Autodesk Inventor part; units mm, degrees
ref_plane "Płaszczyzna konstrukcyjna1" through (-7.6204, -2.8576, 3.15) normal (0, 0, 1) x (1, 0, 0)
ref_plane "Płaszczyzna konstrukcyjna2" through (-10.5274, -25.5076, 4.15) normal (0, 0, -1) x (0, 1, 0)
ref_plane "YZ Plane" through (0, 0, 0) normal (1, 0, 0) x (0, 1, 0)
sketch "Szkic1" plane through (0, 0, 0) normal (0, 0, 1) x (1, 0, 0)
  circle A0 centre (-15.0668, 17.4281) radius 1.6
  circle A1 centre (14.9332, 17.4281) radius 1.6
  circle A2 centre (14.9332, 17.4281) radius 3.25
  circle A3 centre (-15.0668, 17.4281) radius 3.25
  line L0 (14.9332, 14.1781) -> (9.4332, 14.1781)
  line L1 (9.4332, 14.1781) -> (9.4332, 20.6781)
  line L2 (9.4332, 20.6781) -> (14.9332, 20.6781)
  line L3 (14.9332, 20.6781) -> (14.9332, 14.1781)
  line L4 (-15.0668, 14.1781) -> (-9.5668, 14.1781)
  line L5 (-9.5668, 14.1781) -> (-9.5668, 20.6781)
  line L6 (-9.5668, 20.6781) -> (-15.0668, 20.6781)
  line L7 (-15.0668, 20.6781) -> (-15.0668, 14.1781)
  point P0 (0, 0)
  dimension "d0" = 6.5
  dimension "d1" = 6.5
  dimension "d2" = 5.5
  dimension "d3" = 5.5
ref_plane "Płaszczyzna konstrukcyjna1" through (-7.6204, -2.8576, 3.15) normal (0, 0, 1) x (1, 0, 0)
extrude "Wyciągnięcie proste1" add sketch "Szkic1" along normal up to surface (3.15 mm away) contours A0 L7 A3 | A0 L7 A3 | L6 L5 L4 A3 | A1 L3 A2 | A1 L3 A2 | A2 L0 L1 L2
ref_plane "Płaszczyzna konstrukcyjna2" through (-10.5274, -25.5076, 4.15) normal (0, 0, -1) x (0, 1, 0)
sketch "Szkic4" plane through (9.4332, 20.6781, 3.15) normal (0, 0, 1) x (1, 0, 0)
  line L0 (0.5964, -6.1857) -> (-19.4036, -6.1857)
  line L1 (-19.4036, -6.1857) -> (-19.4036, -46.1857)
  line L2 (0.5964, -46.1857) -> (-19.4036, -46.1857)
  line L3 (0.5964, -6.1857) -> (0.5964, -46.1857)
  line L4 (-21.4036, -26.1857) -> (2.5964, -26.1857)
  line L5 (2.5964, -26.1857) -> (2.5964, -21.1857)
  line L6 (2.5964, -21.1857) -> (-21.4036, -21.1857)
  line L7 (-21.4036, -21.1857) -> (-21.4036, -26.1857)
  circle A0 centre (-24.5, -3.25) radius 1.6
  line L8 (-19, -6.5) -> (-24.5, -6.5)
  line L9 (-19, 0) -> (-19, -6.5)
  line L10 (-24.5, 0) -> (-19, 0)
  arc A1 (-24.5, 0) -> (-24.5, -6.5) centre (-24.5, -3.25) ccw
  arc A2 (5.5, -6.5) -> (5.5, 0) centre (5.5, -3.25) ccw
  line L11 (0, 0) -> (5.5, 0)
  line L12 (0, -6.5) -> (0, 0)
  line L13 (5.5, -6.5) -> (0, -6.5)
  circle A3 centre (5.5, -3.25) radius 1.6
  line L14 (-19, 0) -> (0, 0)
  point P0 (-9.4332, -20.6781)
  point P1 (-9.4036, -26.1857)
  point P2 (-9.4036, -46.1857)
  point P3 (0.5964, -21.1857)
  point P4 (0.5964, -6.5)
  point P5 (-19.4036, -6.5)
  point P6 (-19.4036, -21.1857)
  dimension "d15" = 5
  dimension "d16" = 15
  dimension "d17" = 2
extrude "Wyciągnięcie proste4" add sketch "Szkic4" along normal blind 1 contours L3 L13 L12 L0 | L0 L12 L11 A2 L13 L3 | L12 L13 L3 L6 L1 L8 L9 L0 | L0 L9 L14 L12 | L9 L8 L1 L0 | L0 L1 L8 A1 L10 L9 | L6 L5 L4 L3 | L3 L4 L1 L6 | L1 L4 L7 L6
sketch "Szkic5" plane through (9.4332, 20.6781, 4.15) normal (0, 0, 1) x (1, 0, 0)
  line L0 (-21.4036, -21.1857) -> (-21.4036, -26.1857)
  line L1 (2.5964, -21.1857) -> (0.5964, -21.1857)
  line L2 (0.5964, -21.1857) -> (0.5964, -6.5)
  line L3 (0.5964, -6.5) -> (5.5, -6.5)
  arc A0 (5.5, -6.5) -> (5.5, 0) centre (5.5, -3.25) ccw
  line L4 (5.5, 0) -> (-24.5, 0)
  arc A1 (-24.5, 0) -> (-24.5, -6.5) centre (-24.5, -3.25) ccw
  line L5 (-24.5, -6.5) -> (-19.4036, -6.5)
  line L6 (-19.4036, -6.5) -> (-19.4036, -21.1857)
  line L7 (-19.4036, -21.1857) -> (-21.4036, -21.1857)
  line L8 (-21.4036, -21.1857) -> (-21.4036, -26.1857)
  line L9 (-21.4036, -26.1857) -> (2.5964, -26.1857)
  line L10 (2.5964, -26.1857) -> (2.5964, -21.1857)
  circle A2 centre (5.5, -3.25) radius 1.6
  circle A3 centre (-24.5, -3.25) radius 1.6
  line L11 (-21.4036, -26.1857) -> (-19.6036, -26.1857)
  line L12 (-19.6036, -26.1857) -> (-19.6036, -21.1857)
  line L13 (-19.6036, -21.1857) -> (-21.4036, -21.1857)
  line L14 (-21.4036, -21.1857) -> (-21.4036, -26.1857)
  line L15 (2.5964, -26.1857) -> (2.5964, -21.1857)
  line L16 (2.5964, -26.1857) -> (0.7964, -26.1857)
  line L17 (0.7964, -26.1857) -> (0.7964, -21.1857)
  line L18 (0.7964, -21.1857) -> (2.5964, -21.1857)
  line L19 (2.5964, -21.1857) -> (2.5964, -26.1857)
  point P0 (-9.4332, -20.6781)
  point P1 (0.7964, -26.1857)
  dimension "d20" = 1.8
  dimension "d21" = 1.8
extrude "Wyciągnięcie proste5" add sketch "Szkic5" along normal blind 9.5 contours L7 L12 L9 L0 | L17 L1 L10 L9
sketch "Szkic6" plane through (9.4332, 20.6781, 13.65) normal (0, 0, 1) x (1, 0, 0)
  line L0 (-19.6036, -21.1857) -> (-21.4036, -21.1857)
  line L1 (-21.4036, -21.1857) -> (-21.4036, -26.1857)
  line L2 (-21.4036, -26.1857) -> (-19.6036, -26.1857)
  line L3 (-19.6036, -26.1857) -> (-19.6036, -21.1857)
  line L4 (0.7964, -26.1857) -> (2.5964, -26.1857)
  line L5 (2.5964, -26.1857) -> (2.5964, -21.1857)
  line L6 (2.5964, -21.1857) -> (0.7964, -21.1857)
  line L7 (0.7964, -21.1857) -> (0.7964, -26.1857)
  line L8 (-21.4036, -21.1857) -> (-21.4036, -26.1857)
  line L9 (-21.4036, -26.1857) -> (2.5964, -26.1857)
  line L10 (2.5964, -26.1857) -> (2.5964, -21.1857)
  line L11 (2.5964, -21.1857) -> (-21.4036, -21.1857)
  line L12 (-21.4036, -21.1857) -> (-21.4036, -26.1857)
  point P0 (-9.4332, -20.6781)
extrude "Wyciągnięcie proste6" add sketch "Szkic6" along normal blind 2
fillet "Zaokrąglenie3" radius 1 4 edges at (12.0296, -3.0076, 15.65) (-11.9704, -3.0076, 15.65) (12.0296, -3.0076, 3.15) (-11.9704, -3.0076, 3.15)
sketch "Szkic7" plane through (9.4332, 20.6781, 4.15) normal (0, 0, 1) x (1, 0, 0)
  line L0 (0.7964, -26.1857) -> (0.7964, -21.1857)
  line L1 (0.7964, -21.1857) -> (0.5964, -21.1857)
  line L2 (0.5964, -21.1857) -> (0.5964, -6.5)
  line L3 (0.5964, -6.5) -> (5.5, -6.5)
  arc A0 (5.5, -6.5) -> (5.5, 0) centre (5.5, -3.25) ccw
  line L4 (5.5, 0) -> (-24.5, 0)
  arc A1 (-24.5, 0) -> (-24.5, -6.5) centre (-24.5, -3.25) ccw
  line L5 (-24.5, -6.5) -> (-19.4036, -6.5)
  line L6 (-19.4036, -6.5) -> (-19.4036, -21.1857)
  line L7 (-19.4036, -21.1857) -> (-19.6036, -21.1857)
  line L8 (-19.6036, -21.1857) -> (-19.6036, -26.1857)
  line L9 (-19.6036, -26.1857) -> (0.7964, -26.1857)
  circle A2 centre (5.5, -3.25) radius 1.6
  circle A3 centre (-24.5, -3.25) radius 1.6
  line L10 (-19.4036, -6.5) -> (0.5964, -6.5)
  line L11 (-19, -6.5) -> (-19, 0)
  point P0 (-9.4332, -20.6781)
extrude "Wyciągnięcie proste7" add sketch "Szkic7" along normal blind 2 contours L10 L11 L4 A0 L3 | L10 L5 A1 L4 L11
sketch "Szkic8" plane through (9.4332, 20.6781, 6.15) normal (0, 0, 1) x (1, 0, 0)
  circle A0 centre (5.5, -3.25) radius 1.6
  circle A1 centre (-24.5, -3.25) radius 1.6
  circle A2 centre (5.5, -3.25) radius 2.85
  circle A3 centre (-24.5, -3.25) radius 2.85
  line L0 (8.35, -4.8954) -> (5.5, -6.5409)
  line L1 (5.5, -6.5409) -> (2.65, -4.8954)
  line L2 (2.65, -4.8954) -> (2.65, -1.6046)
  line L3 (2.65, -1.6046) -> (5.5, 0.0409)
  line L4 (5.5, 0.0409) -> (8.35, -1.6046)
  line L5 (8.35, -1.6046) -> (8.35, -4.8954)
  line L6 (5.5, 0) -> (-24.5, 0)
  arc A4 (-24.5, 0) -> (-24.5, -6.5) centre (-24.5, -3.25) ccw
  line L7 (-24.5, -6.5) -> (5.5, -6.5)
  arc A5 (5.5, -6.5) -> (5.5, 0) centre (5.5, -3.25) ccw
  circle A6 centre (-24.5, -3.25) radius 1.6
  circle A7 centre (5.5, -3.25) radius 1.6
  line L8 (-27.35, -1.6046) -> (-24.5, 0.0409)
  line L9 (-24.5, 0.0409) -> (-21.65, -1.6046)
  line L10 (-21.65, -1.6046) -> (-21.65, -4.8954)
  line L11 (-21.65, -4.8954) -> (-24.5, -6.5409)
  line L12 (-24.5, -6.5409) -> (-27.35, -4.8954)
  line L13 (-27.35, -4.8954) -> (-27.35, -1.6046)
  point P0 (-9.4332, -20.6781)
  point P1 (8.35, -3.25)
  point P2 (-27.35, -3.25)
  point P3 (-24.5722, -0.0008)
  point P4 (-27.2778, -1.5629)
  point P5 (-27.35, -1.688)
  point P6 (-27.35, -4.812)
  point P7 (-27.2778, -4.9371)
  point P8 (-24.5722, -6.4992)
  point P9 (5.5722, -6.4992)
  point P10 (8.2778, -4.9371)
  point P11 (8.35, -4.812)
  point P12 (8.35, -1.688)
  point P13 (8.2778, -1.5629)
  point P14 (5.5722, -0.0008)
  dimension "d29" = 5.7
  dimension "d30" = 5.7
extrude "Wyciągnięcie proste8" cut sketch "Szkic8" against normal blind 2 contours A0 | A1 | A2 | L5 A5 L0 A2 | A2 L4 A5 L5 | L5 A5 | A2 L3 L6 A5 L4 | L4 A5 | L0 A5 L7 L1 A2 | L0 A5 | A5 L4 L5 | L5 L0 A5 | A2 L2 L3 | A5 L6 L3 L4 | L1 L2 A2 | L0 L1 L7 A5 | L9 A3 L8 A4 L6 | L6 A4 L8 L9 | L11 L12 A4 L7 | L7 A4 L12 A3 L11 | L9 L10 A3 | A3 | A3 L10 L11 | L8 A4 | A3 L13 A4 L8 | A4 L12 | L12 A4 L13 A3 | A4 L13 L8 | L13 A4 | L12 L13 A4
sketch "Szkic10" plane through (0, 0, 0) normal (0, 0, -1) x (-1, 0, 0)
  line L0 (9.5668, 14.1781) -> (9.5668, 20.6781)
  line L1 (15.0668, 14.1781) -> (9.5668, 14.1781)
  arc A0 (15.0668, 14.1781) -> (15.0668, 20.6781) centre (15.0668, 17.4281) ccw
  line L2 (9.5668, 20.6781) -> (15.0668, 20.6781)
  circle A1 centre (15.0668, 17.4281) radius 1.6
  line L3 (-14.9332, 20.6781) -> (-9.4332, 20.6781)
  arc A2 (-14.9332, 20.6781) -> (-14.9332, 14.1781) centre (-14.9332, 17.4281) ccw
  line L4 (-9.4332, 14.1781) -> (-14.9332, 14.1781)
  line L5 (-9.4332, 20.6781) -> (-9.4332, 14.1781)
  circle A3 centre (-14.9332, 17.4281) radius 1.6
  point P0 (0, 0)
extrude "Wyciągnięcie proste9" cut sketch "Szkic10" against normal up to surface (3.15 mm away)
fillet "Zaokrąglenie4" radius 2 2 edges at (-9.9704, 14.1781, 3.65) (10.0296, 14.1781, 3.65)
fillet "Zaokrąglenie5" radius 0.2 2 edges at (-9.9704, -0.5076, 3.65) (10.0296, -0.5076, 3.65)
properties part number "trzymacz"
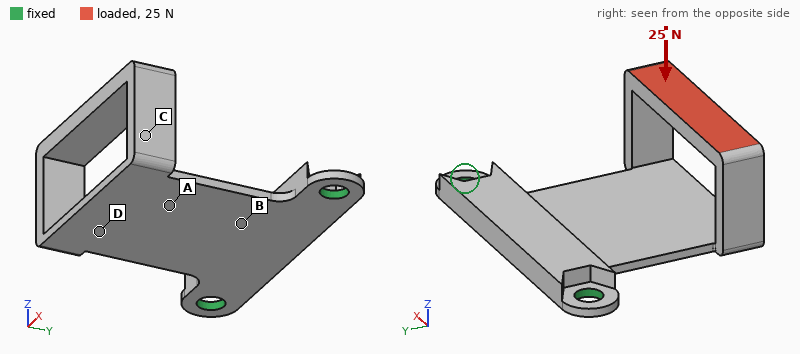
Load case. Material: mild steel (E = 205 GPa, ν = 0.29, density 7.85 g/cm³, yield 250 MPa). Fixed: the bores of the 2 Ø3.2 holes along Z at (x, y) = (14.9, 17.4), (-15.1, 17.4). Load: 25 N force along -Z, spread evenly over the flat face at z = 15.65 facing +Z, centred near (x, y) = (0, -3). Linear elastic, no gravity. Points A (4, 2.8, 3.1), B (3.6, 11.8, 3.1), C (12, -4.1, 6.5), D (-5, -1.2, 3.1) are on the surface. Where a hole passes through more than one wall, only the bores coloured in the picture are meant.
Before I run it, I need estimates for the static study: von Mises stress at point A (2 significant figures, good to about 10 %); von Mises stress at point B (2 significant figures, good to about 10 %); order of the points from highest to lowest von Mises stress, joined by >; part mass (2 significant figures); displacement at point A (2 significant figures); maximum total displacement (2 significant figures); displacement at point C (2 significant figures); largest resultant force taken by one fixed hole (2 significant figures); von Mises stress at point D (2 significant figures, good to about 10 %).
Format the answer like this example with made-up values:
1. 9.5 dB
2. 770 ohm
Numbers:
1. 39 MPa
2. 98 MPa
3. B > A > D > C
4. 11 g
5. 0.087 mm
6. 0.24 mm
7. 0.18 mm
8. 42 N
9. 18 MPa
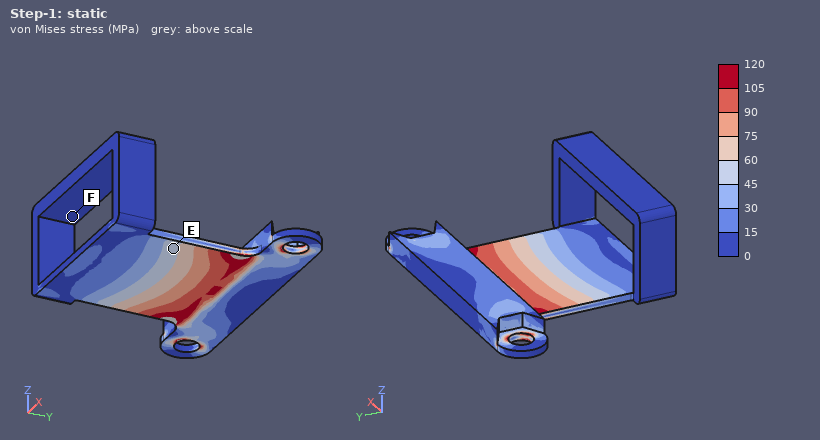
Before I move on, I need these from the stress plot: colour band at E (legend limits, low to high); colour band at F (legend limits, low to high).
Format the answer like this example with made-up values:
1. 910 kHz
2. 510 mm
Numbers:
1. 45 to 60 MPa
2. 0 to 15 MPa
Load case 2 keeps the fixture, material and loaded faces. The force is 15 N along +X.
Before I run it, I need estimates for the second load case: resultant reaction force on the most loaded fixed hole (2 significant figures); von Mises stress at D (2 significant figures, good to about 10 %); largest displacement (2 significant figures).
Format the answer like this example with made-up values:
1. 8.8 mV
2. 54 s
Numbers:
1. 15 N
2. 19 MPa
3. 62 µm
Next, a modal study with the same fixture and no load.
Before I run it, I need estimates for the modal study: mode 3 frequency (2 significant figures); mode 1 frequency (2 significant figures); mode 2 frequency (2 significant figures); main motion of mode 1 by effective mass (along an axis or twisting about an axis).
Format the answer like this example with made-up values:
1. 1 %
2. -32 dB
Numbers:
1. 2400 Hz
2. 790 Hz
3. 1500 Hz
4. along Z
